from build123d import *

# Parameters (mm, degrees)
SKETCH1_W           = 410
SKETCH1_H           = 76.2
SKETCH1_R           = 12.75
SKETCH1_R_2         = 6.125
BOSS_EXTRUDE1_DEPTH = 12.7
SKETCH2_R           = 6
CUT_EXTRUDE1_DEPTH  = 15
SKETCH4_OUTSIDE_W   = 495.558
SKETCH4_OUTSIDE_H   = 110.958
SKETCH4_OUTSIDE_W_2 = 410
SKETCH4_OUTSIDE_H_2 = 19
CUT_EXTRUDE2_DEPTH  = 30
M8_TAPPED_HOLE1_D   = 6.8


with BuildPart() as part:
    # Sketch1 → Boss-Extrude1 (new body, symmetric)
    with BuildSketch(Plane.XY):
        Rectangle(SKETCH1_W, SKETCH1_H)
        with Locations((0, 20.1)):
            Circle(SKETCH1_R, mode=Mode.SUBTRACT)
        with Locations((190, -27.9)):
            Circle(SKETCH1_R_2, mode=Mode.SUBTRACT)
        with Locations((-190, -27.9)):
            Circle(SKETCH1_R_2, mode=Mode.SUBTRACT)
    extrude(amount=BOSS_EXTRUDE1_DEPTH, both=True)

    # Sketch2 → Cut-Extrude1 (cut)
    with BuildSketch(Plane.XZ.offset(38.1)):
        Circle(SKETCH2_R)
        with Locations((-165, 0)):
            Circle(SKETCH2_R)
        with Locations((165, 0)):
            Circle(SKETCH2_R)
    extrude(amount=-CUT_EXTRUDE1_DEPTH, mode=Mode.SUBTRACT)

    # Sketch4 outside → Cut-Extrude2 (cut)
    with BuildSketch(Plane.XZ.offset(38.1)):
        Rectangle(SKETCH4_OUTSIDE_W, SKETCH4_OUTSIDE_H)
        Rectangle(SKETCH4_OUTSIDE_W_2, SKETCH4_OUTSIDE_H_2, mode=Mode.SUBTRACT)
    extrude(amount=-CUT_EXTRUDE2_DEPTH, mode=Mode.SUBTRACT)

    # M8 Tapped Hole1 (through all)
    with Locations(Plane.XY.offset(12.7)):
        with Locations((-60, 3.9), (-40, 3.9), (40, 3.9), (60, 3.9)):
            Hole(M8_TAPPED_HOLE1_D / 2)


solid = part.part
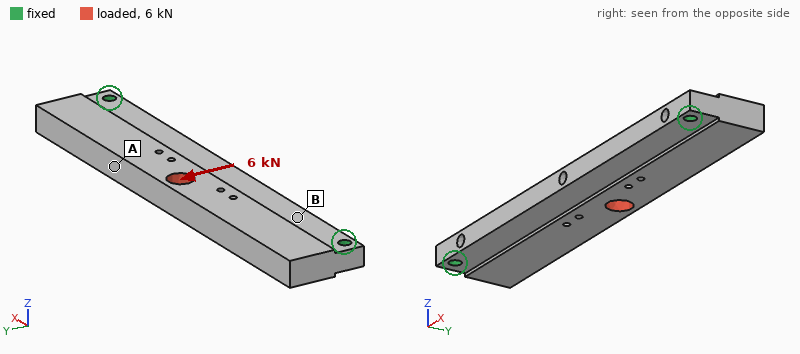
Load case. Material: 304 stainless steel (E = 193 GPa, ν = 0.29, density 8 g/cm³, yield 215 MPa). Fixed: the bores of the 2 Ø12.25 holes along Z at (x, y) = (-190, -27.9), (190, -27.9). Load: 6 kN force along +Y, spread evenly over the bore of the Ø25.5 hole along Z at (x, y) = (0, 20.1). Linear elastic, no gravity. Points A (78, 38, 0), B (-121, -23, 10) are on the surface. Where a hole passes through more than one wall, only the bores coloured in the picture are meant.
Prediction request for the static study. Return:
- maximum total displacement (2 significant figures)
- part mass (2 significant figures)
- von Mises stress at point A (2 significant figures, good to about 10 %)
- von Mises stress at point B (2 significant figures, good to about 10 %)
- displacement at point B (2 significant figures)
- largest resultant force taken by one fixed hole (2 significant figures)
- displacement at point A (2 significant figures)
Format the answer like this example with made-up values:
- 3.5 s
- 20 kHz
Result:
- 33 µm
- 5.5 kg
- 8.3 MPa
- 4.1 MPa
- 13 µm
- 5.7 kN
- 23 µm
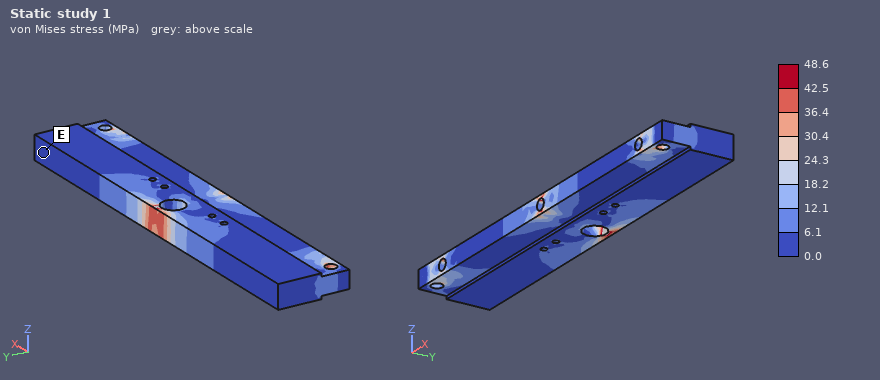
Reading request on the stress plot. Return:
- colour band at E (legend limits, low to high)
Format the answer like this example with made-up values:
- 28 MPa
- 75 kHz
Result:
- 0.0 to 6.1 MPa
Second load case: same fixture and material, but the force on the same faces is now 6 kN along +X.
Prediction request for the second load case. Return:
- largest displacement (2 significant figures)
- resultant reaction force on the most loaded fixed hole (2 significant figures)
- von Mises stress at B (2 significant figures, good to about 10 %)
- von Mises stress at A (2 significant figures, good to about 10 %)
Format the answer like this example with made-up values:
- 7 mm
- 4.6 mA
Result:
- 3.2 µm
- 3.1 kN
- 2.7 MPa
- 1.8 MPa
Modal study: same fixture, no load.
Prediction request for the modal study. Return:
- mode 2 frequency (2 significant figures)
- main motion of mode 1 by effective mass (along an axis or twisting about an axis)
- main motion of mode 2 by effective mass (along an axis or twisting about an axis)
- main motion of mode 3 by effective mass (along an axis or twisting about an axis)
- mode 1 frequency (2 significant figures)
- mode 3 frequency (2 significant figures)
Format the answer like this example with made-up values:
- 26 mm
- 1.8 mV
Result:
- 1500 Hz
- along Z
- along Y
- twisting about X
- 580 Hz
- 1500 Hz
